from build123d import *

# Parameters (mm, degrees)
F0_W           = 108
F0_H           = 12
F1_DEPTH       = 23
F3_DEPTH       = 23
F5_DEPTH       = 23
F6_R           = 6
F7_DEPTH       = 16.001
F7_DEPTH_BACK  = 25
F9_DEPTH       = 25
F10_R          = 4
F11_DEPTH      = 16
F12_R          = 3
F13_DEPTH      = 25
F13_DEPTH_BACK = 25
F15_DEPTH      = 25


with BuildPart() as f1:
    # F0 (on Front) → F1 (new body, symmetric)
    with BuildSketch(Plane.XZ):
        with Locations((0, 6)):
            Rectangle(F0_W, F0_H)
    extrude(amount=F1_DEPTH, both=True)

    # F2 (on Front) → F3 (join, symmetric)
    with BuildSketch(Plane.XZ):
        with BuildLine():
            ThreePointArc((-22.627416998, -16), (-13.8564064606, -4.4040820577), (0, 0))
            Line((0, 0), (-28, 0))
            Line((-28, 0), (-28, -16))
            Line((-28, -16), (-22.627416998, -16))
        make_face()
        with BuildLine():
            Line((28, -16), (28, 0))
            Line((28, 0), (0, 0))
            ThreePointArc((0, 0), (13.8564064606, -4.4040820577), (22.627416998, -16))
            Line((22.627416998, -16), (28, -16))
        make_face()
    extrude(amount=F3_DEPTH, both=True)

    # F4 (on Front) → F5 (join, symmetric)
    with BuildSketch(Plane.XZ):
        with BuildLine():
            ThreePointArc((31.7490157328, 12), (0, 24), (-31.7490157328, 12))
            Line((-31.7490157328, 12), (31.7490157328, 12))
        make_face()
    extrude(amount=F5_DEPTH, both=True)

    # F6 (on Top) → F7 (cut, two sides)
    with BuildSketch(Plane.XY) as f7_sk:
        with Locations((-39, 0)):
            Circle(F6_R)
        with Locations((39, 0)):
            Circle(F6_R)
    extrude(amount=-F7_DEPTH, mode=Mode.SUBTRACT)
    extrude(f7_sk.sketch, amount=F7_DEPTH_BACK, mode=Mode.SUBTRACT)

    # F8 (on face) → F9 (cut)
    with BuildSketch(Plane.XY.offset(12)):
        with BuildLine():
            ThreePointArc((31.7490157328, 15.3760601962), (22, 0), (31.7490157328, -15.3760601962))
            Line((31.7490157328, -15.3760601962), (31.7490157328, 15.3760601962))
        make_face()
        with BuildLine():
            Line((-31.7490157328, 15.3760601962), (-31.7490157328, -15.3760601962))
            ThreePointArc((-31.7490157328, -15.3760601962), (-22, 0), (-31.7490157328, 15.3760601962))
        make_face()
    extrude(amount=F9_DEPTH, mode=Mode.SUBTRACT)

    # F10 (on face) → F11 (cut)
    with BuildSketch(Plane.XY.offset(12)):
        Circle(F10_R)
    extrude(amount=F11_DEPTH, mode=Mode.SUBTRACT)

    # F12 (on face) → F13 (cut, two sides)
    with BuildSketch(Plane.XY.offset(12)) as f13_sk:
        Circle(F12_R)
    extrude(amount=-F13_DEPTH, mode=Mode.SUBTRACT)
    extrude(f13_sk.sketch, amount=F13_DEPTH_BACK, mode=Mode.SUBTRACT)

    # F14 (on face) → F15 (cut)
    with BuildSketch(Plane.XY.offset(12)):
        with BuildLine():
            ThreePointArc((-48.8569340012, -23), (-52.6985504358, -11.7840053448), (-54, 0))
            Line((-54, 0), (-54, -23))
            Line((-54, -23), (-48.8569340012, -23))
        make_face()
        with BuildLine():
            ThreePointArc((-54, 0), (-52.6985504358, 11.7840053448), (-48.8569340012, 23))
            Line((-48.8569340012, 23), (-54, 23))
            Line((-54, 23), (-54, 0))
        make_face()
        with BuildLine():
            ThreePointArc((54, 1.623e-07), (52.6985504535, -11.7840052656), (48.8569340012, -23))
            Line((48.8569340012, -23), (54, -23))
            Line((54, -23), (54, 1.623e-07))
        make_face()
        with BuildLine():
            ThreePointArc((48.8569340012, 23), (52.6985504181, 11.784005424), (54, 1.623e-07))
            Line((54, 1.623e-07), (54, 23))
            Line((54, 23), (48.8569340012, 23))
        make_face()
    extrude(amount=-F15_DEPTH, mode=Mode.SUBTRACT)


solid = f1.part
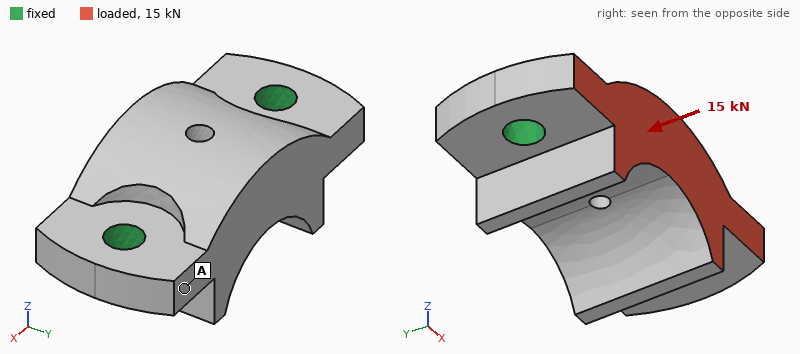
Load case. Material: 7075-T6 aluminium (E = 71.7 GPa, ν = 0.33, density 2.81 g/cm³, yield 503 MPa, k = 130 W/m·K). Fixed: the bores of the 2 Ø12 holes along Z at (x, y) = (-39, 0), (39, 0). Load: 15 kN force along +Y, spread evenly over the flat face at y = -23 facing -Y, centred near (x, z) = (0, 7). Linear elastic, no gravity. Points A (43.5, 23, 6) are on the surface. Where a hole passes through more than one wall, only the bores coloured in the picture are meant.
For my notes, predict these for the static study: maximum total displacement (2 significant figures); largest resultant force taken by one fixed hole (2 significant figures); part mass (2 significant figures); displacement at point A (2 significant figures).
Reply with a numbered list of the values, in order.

1. 19 µm
2. 7.5 kN
3. 260 g
4. 4.3 µm
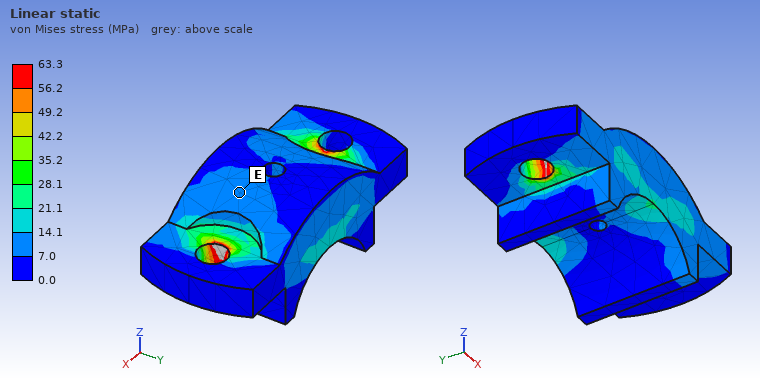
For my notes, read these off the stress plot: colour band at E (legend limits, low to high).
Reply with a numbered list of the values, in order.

1. 7.0 to 14.1 MPa
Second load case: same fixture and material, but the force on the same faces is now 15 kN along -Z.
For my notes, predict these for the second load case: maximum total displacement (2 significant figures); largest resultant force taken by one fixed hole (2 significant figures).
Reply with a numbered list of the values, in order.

1. 0.10 mm
2. 7.6 kN
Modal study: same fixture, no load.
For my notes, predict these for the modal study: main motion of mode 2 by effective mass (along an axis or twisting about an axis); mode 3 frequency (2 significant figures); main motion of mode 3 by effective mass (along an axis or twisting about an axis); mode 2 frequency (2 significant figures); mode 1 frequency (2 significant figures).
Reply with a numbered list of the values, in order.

1. along Z
2. 12 kHz
3. along Y
4. 9100 Hz
5. 7400 Hz
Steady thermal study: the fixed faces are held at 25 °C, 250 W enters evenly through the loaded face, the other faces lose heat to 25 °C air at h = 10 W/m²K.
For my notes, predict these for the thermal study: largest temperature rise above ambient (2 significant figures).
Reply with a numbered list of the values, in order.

1. 44 K
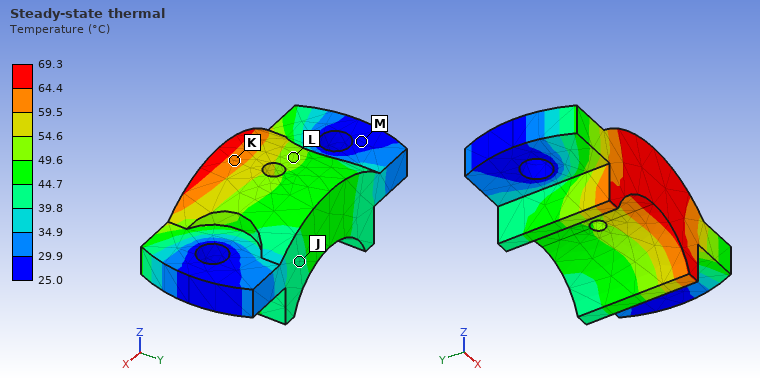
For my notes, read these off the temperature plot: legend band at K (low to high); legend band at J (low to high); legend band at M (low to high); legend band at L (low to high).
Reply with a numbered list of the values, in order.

1. 59.5 to 64.4 °C
2. 39.8 to 44.7 °C
3. 25.0 to 29.9 °C
4. 49.6 to 54.6 °C
